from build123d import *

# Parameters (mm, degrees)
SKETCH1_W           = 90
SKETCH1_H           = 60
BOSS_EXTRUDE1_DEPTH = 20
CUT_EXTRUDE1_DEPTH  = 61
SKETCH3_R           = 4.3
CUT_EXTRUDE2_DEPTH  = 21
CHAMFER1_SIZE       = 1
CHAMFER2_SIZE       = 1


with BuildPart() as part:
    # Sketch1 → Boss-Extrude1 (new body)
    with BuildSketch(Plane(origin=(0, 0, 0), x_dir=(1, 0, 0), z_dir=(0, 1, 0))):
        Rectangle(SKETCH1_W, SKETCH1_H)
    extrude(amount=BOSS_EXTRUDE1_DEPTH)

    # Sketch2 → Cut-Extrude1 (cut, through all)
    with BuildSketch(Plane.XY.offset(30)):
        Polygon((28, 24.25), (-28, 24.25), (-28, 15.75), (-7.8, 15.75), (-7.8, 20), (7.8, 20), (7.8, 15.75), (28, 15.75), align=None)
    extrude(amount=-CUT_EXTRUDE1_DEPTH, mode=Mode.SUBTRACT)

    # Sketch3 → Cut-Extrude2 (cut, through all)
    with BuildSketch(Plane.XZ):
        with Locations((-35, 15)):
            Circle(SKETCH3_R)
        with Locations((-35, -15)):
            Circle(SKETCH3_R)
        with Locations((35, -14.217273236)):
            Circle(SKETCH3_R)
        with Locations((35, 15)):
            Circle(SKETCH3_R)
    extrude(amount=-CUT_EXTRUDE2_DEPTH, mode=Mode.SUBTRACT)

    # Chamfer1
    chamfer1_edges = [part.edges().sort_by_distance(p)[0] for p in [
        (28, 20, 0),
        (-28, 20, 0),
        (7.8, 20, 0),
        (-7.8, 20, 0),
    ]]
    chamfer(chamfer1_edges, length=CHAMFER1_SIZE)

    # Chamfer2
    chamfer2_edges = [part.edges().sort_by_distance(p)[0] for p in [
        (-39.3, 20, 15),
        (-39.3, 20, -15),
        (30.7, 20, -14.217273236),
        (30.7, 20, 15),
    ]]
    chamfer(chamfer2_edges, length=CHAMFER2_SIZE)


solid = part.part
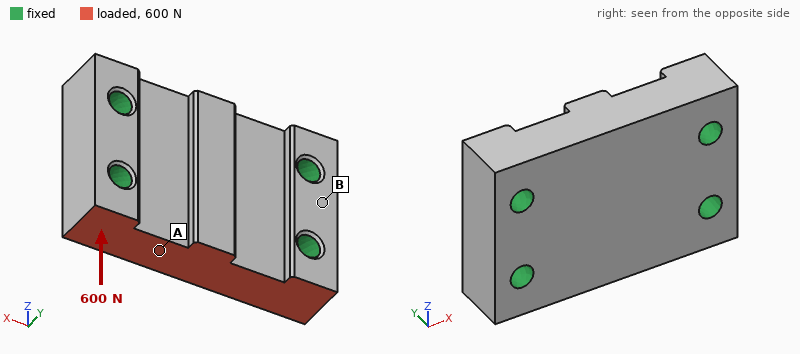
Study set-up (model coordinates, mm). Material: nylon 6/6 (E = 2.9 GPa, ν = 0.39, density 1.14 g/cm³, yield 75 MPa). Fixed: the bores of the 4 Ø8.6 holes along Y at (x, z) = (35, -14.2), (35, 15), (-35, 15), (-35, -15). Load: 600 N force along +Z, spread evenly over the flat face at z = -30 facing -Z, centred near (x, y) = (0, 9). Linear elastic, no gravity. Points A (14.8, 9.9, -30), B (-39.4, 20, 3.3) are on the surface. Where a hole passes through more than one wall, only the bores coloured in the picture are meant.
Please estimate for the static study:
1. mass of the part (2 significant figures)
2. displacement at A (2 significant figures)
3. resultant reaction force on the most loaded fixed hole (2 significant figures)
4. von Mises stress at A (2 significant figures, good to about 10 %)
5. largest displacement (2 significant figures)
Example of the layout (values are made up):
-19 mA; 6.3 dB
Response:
110 g; 5.9 µm; 220 N; 0.36 MPa; 8.0 µm
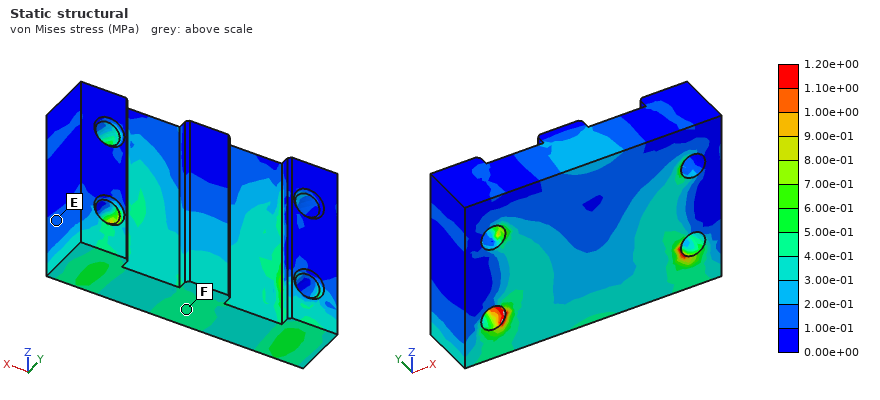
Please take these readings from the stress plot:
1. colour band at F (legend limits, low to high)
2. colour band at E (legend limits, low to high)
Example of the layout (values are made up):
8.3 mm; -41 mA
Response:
4.00e-01 to 5.00e-01 MPa; 1.00e-01 to 2.00e-01 MPa
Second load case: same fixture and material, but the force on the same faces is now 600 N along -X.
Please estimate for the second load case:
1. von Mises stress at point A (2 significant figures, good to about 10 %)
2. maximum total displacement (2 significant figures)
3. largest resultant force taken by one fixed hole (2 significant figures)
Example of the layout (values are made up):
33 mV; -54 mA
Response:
0.64 MPa; 12 µm; 290 N
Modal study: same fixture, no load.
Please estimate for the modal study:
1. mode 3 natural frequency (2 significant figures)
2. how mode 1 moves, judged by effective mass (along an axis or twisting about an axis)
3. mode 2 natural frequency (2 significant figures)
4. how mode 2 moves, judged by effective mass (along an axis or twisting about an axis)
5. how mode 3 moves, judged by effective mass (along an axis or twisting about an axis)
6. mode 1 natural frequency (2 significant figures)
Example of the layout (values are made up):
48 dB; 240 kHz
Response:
5800 Hz; along Y; 4700 Hz; twisting about X; along Z; 4300 Hz
